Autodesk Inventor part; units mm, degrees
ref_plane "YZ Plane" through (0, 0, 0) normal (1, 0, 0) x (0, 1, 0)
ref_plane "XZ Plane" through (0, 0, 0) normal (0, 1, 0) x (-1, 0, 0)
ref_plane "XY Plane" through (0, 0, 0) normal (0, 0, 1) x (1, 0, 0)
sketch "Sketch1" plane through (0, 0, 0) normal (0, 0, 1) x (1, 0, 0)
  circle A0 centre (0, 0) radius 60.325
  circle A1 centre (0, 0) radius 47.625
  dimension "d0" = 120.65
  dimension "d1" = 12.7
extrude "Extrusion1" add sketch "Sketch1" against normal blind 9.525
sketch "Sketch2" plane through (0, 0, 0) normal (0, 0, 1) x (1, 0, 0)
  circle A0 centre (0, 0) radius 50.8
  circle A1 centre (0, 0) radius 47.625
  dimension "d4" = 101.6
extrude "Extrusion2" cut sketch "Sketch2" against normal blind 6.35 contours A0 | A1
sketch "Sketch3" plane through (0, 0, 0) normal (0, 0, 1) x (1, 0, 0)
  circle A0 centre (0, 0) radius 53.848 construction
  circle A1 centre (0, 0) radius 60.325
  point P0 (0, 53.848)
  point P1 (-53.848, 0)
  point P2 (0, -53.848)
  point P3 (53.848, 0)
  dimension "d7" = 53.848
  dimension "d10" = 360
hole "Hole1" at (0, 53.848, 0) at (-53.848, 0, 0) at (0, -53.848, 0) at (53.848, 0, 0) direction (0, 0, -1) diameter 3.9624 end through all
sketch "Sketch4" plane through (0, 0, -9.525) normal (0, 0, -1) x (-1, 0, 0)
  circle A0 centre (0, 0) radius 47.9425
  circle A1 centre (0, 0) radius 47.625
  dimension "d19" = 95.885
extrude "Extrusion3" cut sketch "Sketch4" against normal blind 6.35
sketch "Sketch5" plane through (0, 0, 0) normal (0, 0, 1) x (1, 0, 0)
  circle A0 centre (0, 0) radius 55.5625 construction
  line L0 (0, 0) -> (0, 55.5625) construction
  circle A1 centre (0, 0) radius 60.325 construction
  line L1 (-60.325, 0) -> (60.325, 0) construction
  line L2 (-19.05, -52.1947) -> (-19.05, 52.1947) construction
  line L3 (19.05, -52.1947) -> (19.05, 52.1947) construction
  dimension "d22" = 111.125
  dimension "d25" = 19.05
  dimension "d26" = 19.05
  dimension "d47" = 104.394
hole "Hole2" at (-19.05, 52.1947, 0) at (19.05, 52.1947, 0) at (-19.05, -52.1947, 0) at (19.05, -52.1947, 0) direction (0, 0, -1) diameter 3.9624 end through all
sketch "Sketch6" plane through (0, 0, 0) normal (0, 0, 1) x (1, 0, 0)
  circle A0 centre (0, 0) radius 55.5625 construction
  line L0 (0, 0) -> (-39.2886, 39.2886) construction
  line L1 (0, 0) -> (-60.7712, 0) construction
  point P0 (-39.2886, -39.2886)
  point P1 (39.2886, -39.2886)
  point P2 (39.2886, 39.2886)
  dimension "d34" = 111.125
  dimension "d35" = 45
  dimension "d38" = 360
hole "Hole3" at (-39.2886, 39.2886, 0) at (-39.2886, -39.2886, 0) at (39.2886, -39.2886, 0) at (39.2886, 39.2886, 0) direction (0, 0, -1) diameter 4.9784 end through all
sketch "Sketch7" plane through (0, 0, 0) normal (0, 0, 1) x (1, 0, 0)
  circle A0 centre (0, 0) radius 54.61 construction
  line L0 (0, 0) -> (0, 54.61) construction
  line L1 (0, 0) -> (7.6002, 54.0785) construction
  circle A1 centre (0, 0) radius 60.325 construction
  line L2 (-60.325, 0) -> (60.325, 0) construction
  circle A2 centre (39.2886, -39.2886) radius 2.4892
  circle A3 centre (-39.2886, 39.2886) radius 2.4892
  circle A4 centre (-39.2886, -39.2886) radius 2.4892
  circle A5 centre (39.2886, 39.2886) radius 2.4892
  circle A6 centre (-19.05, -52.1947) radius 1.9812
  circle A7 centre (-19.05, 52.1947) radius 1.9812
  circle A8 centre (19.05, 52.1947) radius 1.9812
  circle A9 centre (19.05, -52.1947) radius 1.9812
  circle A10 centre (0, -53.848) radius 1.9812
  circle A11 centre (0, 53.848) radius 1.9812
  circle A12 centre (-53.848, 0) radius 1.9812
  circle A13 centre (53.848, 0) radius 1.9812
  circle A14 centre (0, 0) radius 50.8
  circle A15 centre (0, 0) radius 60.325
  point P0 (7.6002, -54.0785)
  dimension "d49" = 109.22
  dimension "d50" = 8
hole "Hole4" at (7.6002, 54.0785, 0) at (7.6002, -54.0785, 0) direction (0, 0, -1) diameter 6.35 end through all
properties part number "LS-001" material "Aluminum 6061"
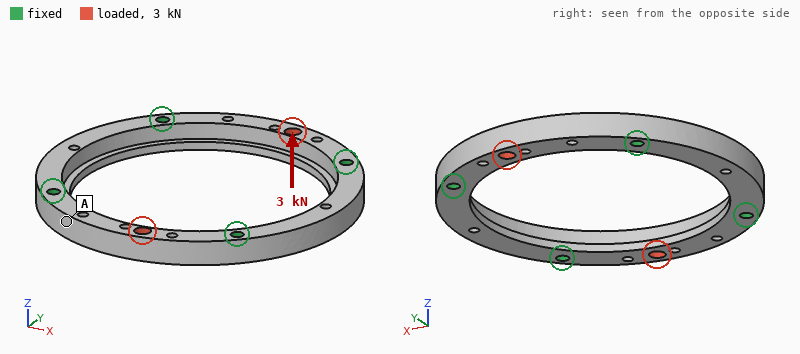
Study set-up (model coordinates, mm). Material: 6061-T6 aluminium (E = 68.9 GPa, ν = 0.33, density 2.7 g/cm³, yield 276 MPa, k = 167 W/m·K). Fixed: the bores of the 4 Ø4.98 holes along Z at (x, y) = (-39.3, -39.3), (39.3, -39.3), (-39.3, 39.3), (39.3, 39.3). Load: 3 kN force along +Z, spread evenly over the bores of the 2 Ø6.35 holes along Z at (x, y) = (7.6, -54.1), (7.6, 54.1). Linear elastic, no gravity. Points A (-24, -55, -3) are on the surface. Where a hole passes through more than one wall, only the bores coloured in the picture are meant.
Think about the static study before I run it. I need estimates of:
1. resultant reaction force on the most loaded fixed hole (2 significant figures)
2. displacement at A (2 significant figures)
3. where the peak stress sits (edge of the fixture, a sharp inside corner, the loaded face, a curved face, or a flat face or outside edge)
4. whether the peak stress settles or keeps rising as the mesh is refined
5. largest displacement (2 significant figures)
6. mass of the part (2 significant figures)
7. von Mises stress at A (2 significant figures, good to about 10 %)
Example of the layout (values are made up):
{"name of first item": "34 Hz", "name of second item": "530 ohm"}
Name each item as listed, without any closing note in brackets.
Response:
{"resultant reaction force on the most loaded fixed hole": "1.0 kN", "displacement at A": "0.047 mm", "where the peak stress sits": "a sharp inside corner", "whether the peak stress settles or keeps rising as the mesh is refined": "keeps rising", "largest displacement": "0.15 mm", "mass of the part": "87 g", "von Mises stress at A": "21 MPa"}
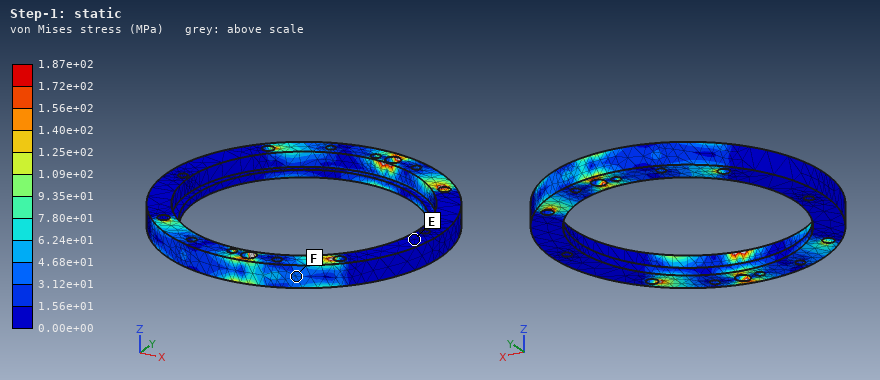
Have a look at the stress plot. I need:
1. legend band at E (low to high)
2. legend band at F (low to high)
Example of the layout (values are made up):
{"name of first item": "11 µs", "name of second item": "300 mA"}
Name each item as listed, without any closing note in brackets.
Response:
{"legend band at E": "0.00e+00 to 1.56e+01 MPa", "legend band at F": "3.12e+01 to 4.68e+01 MPa"}
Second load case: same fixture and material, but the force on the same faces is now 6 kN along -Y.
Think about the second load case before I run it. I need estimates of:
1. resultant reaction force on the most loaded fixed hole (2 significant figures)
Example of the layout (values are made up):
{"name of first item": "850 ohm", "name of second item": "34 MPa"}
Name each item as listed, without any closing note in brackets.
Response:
{"resultant reaction force on the most loaded fixed hole": "2.9 kN"}
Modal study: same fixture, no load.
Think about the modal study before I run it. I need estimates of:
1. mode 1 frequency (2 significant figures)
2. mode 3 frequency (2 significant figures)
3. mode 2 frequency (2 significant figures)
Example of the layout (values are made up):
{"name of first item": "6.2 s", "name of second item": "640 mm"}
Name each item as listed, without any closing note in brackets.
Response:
{"mode 1 frequency": "5900 Hz", "mode 3 frequency": "6100 Hz", "mode 2 frequency": "5900 Hz"}
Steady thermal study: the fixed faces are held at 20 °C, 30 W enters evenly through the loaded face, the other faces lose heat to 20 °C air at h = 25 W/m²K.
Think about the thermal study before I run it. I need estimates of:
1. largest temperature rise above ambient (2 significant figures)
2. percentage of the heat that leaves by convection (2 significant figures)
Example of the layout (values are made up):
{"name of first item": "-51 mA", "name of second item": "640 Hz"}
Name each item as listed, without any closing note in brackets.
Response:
{"largest temperature rise above ambient": "20 K", "percentage of the heat that leaves by convection": "6.0 %"}
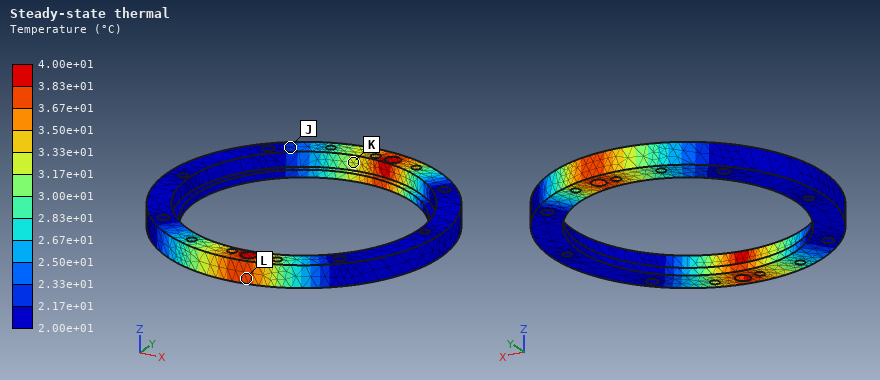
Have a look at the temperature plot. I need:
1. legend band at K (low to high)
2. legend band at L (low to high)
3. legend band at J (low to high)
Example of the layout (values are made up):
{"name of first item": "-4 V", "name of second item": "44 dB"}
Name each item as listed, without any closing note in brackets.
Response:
{"legend band at K": "3.17e+01 to 3.33e+01 °C", "legend band at L": "3.67e+01 to 3.83e+01 °C", "legend band at J": "2.17e+01 to 2.33e+01 °C"}
